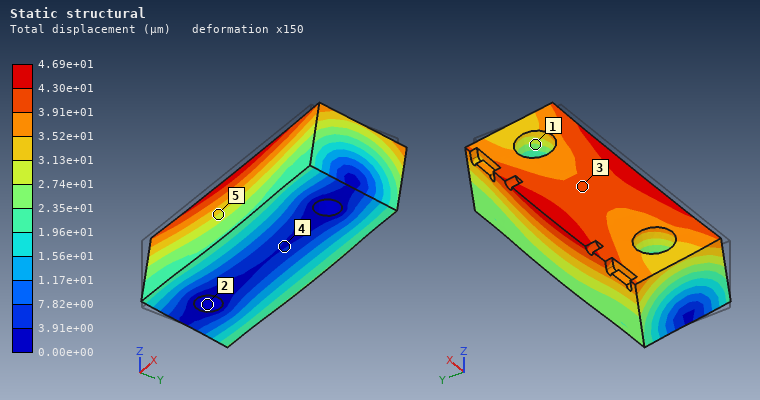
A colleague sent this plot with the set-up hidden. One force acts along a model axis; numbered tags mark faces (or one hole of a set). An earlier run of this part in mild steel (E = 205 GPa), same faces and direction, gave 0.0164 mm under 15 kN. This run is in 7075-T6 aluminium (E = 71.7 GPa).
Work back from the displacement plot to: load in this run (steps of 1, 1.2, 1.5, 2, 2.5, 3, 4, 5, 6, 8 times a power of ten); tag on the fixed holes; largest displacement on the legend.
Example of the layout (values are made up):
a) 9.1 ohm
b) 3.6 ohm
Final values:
a) 15 kN
b) 2
c) 4.69e+01 µm
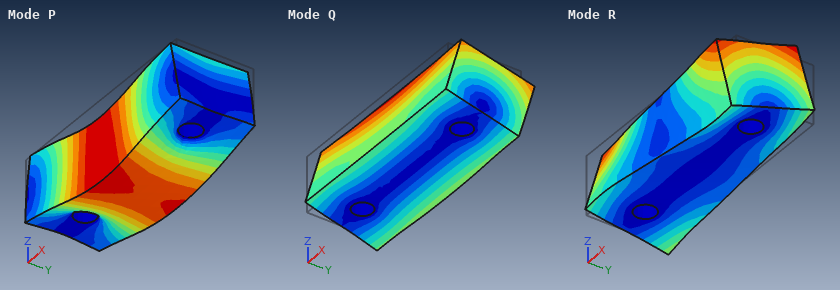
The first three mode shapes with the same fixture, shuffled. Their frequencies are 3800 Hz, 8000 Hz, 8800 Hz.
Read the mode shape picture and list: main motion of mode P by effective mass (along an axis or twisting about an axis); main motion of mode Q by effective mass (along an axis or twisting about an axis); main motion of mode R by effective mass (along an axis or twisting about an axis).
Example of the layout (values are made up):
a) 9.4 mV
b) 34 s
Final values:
a) along Z
b) along Y
c) twisting about Z
